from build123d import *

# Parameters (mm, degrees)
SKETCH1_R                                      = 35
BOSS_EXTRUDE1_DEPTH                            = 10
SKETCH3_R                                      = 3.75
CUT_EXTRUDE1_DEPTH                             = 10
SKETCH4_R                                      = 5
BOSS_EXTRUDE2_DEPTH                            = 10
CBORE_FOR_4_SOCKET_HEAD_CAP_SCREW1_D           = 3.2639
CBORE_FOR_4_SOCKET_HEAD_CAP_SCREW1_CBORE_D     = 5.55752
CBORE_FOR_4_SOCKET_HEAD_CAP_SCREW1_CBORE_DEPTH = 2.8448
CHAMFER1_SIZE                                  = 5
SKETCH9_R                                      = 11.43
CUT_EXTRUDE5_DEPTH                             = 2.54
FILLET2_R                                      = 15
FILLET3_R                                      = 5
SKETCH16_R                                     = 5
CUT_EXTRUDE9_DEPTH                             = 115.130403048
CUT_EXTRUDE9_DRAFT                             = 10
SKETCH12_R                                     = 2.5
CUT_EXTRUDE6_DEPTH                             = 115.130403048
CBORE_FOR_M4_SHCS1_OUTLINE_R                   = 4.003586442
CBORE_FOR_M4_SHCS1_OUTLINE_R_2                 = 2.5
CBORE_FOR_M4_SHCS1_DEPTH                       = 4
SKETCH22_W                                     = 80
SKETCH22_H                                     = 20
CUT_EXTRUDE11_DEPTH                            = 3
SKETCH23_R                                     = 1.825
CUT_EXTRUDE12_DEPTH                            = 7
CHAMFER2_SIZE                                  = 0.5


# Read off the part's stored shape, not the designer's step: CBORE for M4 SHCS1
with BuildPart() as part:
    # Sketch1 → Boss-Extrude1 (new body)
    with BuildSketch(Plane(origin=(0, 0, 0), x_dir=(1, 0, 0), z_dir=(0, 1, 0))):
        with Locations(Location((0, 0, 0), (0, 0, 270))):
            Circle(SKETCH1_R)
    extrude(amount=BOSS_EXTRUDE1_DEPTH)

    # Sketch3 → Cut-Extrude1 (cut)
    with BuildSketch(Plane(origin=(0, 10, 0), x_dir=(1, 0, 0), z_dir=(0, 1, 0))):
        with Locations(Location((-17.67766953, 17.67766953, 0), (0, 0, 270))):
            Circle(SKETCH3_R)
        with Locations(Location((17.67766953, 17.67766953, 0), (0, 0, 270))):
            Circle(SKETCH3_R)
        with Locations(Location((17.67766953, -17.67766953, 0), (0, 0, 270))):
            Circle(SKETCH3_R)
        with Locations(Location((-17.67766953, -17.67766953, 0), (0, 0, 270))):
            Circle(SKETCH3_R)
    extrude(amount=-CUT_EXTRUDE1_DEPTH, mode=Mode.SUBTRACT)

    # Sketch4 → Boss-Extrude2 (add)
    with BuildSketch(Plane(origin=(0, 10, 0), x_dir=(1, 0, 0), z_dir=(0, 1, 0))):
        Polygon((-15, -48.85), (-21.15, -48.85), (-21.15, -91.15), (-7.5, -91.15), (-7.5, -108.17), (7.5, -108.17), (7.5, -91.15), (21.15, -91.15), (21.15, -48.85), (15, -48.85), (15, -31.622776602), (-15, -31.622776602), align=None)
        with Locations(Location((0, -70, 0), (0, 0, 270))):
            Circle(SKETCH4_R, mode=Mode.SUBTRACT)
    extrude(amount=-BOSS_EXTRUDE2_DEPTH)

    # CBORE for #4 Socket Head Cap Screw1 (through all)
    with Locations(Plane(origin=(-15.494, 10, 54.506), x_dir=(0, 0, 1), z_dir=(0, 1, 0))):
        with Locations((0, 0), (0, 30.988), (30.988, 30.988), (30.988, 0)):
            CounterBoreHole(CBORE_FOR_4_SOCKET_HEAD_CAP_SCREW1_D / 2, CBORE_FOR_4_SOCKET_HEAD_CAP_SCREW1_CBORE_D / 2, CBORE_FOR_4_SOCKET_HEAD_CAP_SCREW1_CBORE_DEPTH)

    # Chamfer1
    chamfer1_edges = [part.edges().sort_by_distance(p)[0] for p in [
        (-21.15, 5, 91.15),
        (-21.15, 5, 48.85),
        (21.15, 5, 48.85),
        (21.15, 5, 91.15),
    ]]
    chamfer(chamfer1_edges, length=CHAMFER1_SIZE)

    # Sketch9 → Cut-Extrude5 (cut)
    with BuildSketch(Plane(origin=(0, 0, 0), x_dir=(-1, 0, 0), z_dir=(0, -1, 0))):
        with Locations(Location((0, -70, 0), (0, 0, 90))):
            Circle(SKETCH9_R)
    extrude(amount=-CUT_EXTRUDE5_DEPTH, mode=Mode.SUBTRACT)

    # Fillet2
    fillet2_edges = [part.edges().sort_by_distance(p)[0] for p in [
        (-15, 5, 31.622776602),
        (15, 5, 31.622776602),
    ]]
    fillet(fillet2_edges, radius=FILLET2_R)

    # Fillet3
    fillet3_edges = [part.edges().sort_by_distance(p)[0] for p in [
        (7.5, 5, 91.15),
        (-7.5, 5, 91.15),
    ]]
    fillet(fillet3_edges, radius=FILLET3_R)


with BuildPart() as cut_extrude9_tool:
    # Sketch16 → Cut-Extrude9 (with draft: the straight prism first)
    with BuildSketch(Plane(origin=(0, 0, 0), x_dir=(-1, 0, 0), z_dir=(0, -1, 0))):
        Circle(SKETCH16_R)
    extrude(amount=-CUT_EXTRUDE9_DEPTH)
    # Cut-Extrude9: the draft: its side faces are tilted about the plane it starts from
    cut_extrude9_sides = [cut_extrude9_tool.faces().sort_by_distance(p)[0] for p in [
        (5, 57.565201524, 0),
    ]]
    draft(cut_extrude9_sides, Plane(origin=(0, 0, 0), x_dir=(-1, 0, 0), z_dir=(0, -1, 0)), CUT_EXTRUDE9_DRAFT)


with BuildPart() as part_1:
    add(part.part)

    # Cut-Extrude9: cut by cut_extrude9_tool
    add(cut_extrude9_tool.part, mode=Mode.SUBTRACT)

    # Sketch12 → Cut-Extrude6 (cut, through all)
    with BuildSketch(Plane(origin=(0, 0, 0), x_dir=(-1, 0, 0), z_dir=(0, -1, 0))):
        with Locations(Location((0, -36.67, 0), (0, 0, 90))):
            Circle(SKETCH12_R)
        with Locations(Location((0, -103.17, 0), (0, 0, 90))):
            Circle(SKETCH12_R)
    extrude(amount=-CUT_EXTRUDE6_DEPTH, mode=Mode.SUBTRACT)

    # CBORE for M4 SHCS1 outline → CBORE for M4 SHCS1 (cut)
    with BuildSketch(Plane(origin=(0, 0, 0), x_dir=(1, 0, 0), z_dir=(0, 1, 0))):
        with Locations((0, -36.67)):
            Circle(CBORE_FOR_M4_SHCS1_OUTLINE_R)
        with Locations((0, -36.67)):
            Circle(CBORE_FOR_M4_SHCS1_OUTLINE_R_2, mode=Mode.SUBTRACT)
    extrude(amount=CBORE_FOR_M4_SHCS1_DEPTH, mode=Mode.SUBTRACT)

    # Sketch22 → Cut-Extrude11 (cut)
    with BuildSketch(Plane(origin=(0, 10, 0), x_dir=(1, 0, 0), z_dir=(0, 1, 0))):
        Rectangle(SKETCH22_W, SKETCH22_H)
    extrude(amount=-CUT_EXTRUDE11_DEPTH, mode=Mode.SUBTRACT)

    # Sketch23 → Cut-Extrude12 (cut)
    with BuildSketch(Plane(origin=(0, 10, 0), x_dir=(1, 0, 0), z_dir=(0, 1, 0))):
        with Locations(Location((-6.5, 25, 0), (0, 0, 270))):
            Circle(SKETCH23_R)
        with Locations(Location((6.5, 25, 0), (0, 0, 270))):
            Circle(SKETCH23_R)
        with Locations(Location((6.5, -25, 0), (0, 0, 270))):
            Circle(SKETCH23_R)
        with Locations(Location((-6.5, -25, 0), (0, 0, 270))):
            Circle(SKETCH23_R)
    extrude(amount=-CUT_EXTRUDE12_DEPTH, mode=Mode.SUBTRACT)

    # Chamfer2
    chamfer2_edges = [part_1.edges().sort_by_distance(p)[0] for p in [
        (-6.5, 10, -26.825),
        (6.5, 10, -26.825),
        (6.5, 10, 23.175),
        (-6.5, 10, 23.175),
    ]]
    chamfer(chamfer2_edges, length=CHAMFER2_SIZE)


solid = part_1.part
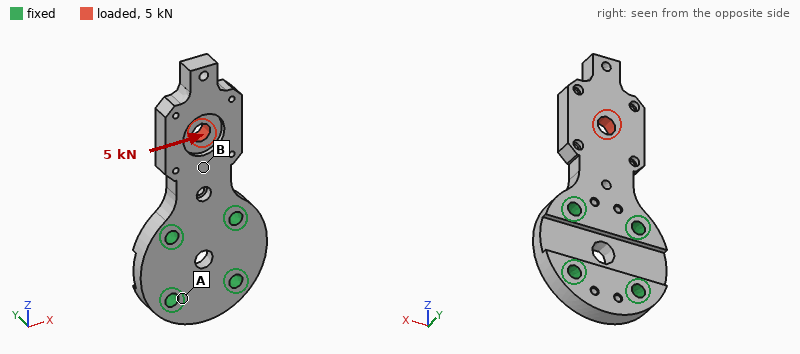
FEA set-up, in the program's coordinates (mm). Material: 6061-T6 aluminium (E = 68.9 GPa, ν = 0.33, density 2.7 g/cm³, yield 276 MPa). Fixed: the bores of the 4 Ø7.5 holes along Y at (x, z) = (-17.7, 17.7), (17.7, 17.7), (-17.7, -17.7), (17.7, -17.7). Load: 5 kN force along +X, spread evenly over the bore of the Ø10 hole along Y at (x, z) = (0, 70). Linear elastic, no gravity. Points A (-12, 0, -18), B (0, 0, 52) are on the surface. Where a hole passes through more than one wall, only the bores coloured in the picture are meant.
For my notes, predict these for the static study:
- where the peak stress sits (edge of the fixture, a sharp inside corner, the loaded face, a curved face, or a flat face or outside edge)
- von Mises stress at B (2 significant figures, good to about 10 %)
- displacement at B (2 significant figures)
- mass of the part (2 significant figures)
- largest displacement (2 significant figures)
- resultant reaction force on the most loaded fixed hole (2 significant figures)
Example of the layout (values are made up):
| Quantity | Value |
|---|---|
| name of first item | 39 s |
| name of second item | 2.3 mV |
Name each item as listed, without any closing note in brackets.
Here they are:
| Quantity | Value |
|---|---|
| where the peak stress sits | a curved face |
| von Mises stress at B | 47 MPa |
| displacement at B | 0.051 mm |
| mass of the part | 140 g |
| largest displacement | 0.24 mm |
| resultant reaction force on the most loaded fixed hole | 7.2 kN |
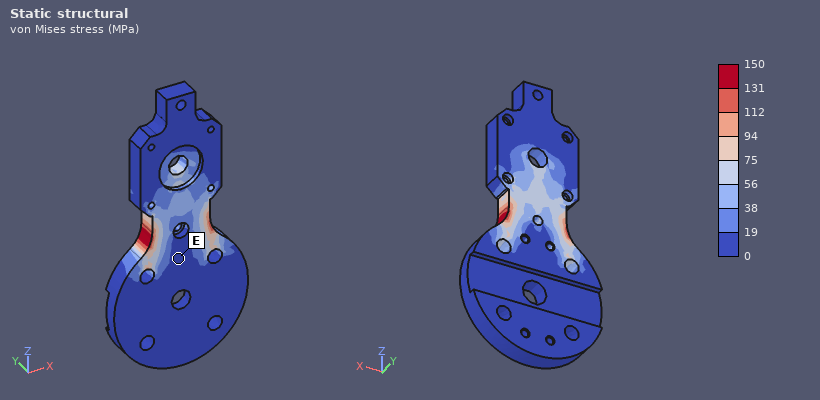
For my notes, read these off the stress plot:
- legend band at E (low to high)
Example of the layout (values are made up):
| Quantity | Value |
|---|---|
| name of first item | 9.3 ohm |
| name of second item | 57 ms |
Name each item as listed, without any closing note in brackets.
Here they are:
| Quantity | Value |
|---|---|
| legend band at E | 0 to 19 MPa |
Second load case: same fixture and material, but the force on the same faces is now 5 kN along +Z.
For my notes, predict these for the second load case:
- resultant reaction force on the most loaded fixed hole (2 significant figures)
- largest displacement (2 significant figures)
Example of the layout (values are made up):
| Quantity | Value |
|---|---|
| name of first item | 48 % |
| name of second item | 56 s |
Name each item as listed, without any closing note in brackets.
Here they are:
| Quantity | Value |
|---|---|
| resultant reaction force on the most loaded fixed hole | 2.4 kN |
| largest displacement | 0.11 mm |
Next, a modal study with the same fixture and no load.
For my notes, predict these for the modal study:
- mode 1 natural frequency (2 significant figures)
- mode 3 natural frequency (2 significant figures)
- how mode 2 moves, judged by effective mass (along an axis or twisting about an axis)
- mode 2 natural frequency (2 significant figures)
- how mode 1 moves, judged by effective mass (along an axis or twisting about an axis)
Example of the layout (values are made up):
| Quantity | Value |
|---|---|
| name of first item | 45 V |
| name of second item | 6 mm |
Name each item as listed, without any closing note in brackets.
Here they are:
| Quantity | Value |
|---|---|
| mode 1 natural frequency | 1200 Hz |
| mode 3 natural frequency | 4500 Hz |
| how mode 2 moves, judged by effective mass | along X |
| mode 2 natural frequency | 3700 Hz |
| how mode 1 moves, judged by effective mass | along Y |
